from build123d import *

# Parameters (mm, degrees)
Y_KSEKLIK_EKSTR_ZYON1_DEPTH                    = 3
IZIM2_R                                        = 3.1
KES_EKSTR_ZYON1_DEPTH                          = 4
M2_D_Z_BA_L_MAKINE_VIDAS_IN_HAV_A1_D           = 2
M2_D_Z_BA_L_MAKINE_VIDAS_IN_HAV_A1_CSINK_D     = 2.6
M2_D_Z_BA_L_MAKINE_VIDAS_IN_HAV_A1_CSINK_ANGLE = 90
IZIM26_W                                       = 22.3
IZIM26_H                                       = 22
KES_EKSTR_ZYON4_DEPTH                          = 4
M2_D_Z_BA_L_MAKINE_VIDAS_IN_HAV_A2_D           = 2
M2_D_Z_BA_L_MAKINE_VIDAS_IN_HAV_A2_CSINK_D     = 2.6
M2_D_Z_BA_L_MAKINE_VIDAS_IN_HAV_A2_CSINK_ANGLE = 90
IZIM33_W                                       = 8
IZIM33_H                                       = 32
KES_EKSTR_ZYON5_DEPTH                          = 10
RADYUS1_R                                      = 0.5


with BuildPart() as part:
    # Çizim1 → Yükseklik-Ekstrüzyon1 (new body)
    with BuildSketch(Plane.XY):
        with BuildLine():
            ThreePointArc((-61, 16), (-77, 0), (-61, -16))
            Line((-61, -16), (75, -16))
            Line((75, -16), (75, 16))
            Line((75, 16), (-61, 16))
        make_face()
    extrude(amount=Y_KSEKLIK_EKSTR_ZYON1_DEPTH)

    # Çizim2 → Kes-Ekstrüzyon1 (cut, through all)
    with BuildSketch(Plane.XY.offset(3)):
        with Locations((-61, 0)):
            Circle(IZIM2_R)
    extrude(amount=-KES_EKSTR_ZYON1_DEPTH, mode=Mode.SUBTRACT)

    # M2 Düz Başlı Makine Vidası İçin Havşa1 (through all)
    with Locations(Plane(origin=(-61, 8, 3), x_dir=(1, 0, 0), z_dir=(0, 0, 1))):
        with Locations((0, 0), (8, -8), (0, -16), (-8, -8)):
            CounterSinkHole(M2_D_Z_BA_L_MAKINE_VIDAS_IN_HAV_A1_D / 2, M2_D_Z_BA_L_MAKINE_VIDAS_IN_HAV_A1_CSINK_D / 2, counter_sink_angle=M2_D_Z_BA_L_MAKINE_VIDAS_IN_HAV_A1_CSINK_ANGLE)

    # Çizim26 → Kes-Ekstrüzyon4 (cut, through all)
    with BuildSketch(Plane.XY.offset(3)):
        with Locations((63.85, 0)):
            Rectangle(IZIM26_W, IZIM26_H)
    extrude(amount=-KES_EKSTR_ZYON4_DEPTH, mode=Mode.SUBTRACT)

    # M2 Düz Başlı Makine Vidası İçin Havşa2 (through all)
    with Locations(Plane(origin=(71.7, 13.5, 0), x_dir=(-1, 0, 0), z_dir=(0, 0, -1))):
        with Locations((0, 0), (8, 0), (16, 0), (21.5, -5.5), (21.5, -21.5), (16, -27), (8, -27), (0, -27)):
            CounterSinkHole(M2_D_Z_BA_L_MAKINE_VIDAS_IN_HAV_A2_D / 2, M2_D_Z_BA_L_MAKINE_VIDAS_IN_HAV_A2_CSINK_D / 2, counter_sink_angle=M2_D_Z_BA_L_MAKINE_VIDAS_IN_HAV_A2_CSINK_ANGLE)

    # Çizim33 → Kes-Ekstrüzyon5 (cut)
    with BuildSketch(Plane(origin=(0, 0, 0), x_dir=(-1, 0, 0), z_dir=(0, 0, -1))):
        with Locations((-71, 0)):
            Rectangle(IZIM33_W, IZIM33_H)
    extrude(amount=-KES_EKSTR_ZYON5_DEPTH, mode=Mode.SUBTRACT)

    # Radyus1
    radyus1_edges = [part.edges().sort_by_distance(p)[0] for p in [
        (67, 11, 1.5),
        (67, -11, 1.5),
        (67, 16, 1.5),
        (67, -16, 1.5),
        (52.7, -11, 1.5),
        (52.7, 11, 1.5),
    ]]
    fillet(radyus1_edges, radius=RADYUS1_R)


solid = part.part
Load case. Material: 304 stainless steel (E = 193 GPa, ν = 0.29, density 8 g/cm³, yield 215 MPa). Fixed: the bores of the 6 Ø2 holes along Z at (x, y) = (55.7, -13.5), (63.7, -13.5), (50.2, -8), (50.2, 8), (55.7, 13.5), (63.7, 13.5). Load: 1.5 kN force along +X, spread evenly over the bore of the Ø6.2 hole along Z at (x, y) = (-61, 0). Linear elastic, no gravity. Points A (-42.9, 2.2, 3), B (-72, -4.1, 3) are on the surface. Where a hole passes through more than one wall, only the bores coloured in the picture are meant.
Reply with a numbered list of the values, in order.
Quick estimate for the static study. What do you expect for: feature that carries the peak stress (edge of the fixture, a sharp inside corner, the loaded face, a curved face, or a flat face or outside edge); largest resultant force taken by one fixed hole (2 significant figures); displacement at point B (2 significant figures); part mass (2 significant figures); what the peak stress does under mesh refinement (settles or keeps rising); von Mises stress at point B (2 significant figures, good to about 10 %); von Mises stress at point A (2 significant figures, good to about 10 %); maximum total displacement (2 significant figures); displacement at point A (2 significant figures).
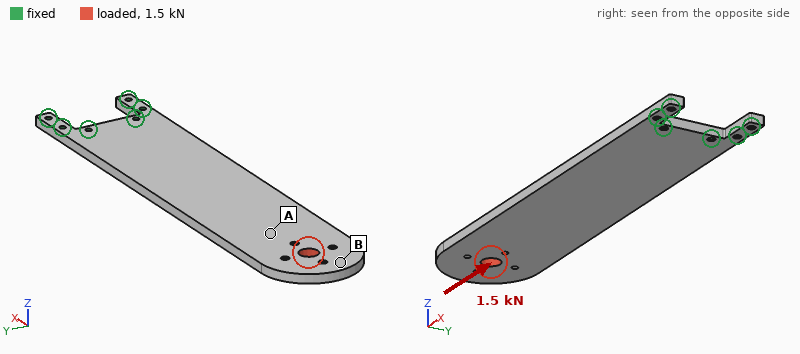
1. edge of the fixture
2. 550 N
3. 10 µm
4. 99 g
5. keeps rising
6. 10.0 MPa
7. 18 MPa
8. 11 µm
9. 8.0 µm
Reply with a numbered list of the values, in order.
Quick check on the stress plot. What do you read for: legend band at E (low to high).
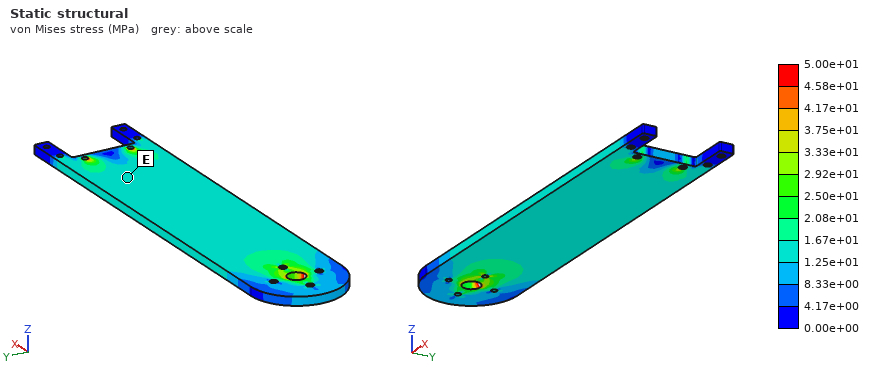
1. 1.25e+01 to 1.67e+01 MPa
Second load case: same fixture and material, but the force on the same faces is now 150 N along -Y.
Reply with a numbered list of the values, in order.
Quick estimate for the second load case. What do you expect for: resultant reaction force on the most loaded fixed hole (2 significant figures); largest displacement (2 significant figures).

1. 450 N
2. 60 µm
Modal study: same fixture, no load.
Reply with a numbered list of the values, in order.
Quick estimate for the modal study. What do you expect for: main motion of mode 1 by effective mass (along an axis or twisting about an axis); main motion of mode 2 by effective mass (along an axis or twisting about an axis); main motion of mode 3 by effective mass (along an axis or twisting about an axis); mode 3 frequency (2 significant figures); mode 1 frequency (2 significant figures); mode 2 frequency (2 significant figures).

1. along Z
2. along Z
3. twisting about X
4. 1200 Hz
5. 160 Hz
6. 960 Hz
